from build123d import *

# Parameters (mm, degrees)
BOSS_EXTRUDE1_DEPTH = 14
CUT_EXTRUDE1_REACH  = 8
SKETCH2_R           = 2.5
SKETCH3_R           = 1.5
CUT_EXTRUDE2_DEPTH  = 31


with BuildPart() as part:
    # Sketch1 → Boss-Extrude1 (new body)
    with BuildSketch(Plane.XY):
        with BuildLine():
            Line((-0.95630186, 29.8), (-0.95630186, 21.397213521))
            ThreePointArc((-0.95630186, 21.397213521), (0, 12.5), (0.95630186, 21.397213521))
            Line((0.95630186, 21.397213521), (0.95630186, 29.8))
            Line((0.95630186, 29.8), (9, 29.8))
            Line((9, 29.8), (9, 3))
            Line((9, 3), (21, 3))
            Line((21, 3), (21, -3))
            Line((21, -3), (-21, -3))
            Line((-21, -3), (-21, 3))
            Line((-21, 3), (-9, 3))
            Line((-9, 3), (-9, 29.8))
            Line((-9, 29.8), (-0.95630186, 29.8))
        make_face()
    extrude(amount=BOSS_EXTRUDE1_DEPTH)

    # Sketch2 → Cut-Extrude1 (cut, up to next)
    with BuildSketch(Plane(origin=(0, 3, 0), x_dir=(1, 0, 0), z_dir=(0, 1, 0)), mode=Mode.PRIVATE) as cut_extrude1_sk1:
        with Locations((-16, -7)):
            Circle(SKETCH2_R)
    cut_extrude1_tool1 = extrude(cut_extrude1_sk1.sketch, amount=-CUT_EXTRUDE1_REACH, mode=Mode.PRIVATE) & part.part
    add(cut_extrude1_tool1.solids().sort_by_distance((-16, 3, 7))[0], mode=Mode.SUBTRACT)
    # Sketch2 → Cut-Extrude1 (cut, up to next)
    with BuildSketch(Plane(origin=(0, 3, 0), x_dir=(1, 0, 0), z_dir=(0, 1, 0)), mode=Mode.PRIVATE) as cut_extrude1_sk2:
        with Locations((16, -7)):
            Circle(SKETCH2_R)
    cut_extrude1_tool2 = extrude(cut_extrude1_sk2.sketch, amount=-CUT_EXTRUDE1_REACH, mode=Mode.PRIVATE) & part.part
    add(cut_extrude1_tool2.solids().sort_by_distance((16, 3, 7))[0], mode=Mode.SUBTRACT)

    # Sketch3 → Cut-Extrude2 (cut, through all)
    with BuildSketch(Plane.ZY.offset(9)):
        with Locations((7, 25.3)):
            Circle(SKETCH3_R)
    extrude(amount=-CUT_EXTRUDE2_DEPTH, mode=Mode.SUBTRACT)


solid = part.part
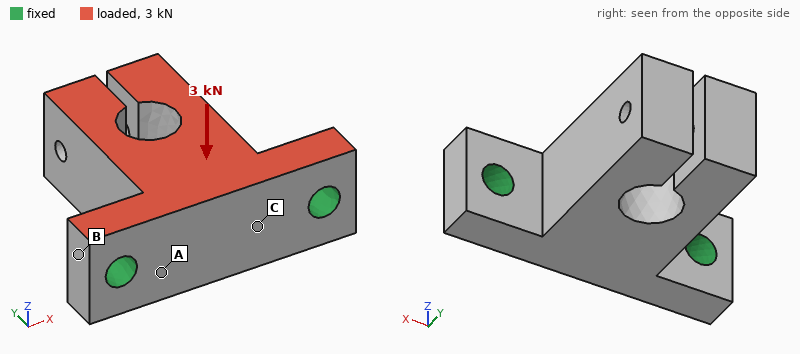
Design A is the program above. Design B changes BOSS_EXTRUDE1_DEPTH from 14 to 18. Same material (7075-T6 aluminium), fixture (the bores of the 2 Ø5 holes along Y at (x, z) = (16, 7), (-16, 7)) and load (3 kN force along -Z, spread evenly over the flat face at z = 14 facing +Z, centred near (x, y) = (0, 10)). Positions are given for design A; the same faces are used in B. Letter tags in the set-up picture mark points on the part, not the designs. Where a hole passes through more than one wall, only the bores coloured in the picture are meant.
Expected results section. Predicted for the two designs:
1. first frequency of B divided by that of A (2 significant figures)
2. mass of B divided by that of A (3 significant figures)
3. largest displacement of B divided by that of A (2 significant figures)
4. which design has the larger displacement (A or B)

1.00
1.30
0.76
A
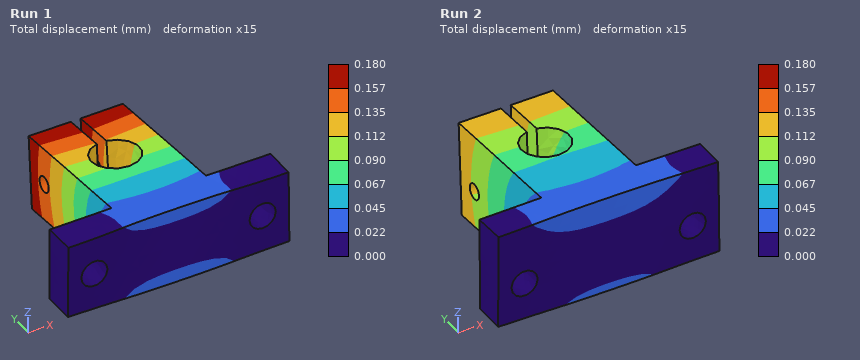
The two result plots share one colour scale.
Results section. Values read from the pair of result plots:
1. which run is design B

Run 2
